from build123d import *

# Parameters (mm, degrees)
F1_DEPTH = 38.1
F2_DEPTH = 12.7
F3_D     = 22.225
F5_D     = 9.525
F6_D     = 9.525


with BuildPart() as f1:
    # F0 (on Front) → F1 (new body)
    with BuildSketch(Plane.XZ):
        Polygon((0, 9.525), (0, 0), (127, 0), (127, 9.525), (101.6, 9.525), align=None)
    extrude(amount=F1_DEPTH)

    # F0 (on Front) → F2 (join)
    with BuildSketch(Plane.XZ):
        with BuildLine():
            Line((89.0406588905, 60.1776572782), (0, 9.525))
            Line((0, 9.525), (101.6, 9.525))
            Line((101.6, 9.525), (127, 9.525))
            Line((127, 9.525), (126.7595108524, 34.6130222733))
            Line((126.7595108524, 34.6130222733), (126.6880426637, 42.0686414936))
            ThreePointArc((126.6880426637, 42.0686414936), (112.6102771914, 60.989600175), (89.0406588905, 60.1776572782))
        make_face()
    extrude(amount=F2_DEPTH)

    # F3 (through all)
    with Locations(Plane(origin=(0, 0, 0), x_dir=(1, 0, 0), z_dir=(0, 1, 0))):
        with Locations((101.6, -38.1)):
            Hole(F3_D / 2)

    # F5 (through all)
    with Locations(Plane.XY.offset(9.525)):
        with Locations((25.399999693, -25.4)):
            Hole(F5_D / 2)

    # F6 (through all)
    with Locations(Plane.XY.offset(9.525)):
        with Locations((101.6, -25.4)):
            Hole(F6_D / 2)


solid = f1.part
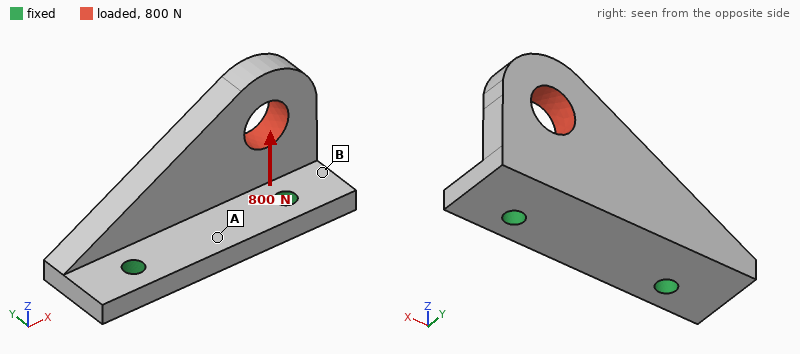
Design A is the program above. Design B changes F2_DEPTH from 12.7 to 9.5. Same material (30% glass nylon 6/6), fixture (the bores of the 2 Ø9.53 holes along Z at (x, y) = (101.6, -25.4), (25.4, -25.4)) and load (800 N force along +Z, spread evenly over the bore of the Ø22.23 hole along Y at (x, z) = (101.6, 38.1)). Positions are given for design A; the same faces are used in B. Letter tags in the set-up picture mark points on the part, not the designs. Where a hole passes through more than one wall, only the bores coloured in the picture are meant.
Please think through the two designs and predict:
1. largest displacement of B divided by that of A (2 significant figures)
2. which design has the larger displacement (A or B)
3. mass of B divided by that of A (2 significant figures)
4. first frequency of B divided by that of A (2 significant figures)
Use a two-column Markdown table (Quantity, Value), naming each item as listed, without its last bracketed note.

| Quantity | Value |
|---|---|
| largest displacement of B divided by that of A | 1.3 |
| which design has the larger displacement | B |
| mass of B divided by that of A | 0.87 |
| first frequency of B divided by that of A | 0.98 |
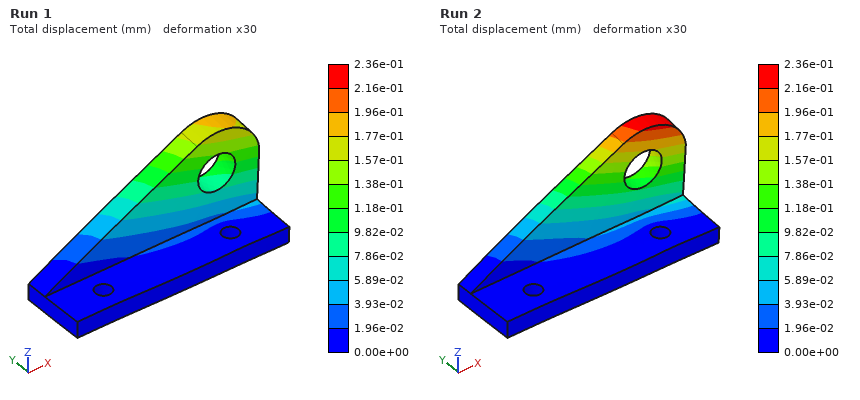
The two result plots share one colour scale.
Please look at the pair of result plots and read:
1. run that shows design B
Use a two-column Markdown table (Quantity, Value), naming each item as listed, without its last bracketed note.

| Quantity | Value |
|---|---|
| run that shows design B | Run 2 |
